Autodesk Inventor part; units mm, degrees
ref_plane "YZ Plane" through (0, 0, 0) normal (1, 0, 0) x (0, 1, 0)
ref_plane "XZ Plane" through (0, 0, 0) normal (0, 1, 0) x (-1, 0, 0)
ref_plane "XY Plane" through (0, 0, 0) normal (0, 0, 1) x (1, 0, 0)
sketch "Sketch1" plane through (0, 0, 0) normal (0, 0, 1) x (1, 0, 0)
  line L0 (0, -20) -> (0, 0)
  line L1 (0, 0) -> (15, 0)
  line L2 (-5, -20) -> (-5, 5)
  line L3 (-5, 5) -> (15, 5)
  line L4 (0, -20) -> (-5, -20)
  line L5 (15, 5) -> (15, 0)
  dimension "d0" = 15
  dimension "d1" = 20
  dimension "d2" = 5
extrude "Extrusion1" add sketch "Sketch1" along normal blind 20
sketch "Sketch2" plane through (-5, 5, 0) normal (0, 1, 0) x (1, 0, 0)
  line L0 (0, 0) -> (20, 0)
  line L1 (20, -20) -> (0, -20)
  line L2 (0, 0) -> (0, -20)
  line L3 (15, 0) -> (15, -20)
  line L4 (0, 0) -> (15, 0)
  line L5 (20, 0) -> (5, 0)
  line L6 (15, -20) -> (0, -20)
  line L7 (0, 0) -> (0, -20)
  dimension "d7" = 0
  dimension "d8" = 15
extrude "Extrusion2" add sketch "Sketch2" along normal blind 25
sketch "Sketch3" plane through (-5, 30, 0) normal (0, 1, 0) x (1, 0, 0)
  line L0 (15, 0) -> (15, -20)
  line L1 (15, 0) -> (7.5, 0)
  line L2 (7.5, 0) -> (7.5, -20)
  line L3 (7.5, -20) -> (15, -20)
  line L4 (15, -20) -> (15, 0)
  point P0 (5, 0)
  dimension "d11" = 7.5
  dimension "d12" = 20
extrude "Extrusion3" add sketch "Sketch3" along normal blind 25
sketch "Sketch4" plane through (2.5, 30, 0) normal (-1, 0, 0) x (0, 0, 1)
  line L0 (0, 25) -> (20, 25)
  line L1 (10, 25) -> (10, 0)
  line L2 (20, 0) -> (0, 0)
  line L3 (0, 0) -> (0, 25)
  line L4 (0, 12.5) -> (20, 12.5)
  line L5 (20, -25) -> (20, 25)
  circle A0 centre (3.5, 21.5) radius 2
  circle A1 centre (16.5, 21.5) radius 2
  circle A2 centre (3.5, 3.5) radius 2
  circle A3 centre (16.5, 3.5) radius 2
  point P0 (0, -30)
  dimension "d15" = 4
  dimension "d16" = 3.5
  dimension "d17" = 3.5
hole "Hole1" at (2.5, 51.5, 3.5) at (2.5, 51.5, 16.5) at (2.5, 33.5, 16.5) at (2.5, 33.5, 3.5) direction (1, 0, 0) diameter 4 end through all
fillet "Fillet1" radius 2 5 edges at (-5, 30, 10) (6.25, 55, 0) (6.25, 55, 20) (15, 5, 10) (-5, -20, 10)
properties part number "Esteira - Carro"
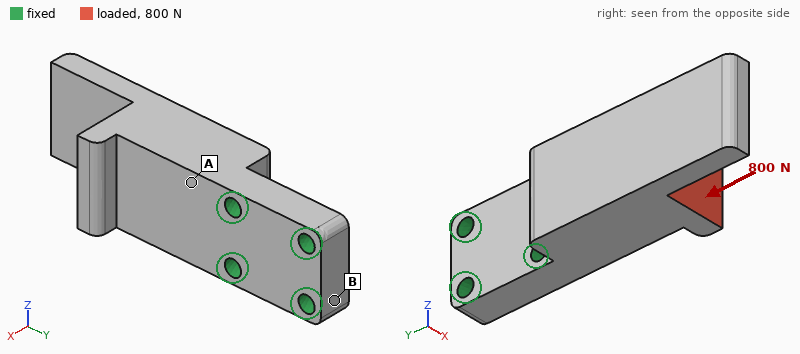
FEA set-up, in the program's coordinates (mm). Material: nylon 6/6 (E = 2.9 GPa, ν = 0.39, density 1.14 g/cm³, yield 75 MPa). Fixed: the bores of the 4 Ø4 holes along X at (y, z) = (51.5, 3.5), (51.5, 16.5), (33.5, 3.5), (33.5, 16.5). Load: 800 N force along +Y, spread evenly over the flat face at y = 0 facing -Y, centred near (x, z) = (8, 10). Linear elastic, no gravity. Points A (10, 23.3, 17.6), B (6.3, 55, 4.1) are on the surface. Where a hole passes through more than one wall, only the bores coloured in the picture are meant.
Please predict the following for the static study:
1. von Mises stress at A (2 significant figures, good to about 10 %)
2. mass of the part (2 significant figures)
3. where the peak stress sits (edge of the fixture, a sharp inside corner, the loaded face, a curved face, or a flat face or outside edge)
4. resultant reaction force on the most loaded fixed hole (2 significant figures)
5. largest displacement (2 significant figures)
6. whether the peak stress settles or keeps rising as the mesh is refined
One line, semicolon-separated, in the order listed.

8.8 MPa; 17 g; edge of the fixture; 390 N; 0.36 mm; keeps rising
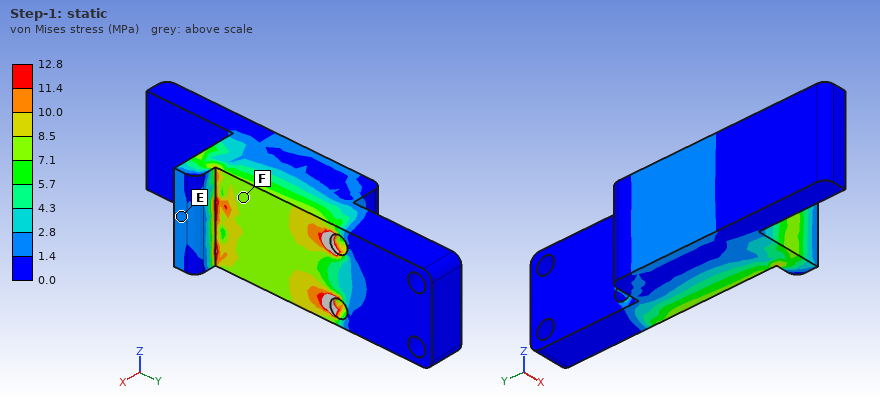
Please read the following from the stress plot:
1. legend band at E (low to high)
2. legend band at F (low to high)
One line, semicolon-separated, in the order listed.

1.4 to 2.8 MPa; 7.1 to 8.5 MPa
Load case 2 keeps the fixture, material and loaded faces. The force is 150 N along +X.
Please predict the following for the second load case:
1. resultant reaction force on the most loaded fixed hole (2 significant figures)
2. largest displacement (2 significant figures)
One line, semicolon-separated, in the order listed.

92 N; 0.80 mm
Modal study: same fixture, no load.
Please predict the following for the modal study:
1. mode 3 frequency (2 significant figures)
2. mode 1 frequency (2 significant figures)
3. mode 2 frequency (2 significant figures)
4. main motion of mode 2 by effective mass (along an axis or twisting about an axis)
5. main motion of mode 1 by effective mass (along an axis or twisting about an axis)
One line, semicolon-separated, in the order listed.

3200 Hz; 950 Hz; 2000 Hz; along Z; along X
